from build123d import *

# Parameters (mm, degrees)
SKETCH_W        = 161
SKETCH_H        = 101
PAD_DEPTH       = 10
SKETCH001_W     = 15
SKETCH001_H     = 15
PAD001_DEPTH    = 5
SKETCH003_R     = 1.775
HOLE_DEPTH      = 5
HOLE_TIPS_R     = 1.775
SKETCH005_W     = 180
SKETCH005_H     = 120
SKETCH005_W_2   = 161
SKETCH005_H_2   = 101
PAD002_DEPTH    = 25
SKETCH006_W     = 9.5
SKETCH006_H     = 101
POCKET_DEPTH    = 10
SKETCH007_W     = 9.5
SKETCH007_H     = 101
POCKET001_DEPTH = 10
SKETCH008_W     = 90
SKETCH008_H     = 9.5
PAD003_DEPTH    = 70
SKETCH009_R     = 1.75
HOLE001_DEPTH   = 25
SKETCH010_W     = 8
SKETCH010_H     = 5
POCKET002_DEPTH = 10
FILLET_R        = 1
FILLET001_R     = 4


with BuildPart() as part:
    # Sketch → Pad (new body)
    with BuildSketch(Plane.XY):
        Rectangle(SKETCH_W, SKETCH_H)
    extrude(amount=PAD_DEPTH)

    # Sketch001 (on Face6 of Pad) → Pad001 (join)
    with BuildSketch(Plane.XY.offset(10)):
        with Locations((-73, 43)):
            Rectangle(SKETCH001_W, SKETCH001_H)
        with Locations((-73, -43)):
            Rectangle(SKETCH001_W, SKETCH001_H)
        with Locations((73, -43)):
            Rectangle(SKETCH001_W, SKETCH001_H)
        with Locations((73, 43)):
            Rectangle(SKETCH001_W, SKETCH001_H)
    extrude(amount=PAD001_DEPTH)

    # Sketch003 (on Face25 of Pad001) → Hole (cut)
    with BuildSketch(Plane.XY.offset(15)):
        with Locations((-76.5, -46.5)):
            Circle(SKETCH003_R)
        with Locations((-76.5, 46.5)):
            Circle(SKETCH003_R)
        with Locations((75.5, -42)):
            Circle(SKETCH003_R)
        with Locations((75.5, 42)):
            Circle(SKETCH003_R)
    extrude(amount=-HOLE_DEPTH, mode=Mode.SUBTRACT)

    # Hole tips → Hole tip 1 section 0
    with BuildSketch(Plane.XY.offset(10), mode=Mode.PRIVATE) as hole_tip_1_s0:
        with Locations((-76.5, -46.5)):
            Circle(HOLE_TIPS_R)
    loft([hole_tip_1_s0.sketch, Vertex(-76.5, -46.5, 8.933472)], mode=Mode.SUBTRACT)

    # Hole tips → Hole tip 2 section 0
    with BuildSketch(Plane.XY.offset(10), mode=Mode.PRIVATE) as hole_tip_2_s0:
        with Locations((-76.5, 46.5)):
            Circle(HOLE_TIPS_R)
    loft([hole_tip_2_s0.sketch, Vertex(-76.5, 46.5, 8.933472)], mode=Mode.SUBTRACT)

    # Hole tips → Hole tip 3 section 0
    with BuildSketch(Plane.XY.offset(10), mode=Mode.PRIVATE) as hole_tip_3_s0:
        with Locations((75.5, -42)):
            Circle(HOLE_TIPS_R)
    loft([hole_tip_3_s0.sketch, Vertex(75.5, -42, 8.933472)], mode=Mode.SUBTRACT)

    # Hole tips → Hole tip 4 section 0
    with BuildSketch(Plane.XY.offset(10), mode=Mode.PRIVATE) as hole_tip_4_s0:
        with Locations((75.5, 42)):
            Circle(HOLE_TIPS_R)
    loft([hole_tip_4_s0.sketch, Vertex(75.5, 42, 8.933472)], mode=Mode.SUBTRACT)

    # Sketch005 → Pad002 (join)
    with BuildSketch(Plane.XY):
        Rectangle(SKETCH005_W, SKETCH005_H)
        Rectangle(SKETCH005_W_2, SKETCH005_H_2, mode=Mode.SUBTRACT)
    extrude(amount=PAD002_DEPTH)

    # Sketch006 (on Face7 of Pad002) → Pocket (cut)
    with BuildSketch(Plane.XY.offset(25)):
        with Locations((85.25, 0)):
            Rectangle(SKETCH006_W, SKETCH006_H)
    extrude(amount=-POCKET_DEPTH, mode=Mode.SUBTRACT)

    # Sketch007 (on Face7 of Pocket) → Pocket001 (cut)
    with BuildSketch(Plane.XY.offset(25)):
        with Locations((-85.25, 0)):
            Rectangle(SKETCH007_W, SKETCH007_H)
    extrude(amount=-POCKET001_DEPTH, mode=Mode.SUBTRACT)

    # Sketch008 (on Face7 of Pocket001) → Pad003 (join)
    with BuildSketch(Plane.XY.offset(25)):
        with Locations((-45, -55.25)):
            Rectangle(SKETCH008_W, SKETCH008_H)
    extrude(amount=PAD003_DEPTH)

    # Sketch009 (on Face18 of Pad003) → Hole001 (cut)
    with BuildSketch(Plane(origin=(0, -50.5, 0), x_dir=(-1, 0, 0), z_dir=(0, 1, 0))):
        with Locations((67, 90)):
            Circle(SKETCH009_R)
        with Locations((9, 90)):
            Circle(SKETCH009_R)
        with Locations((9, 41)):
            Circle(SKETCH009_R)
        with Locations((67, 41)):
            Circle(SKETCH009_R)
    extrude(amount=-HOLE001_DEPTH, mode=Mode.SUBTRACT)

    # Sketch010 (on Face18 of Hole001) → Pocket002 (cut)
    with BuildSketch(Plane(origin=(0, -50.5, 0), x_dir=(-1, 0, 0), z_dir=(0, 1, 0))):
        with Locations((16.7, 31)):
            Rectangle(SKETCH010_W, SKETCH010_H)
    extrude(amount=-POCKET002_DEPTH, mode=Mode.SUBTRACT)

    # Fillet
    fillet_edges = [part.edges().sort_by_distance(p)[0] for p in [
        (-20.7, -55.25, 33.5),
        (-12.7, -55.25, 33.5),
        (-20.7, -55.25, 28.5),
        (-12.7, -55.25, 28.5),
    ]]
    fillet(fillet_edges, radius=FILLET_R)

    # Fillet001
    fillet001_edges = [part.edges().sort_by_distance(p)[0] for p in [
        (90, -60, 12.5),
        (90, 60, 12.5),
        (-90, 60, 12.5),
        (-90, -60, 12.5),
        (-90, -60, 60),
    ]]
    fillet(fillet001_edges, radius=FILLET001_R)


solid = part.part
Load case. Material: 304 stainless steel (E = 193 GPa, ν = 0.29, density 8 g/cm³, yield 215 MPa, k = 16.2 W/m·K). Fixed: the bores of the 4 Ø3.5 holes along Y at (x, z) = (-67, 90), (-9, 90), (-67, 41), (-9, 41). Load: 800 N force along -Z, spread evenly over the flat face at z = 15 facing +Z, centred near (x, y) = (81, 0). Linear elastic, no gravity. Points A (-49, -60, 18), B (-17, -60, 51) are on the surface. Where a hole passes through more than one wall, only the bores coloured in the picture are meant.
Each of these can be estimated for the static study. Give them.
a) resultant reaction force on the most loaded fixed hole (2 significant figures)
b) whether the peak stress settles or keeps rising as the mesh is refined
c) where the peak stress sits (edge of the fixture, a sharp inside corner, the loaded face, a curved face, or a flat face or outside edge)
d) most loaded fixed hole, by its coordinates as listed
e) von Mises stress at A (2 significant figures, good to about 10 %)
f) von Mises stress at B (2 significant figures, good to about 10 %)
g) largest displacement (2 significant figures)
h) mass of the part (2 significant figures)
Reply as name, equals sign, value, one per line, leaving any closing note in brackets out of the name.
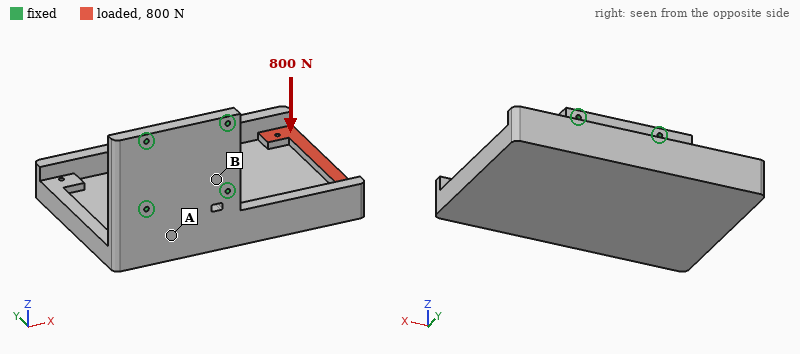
resultant reaction force on the most loaded fixed hole = 1.7 kN
whether the peak stress settles or keeps rising as the mesh is refined = keeps rising
where the peak stress sits = edge of the fixture
most loaded fixed hole, by its coordinates as listed = (-9, 41)
von Mises stress at A = 27 MPa
von Mises stress at B = 8.4 MPa
largest displacement = 0.37 mm
mass of the part = 2.7 kg
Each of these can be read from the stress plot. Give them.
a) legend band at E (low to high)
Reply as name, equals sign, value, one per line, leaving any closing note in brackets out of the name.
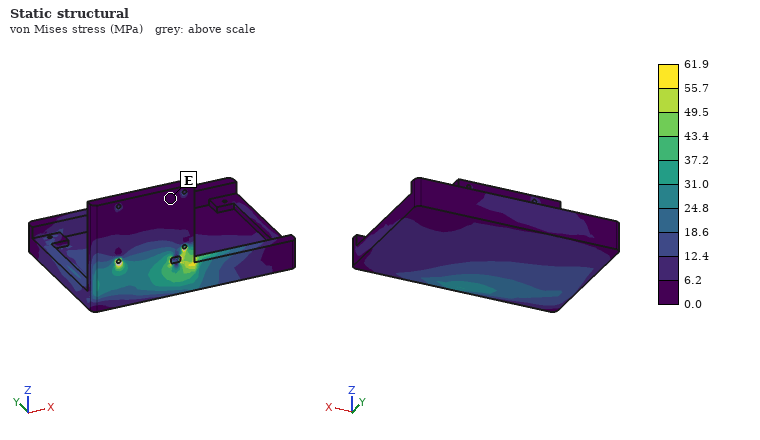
legend band at E = 0.0 to 6.2 MPa
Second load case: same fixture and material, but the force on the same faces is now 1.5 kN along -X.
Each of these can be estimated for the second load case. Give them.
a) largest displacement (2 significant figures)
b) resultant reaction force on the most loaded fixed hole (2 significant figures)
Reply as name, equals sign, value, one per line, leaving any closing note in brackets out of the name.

largest displacement = 0.12 mm
resultant reaction force on the most loaded fixed hole = 1.7 kN
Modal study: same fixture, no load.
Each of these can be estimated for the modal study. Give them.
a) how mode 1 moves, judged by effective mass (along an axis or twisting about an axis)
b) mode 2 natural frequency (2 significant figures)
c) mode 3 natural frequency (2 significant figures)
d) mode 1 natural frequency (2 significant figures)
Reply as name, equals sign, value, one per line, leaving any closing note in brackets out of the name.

how mode 1 moves, judged by effective mass = along Z
mode 2 natural frequency = 430 Hz
mode 3 natural frequency = 700 Hz
mode 1 natural frequency = 230 Hz
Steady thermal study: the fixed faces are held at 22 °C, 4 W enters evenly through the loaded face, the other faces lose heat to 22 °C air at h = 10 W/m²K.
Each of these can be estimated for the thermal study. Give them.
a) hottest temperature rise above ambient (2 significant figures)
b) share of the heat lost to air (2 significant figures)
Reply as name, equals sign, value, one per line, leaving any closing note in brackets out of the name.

hottest temperature rise above ambient = 14 K
share of the heat lost to air = 84 %
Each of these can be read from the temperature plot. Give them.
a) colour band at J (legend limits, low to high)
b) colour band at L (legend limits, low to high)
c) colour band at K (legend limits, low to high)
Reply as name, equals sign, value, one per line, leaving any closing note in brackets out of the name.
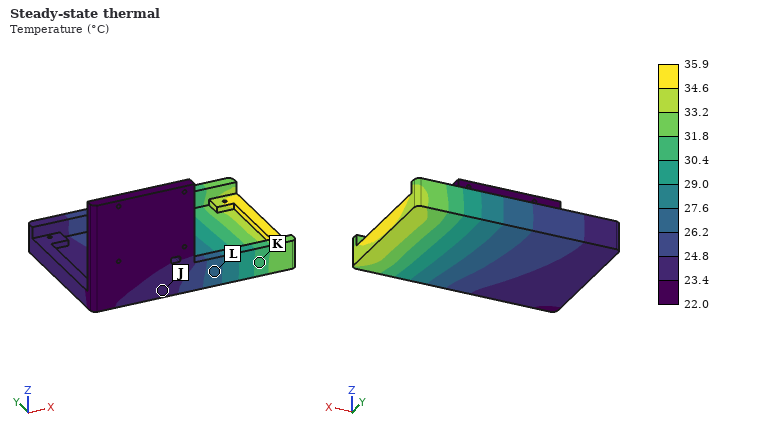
colour band at J = 23.4 to 24.8 °C
colour band at L = 26.2 to 27.6 °C
colour band at K = 30.4 to 31.8 °C
